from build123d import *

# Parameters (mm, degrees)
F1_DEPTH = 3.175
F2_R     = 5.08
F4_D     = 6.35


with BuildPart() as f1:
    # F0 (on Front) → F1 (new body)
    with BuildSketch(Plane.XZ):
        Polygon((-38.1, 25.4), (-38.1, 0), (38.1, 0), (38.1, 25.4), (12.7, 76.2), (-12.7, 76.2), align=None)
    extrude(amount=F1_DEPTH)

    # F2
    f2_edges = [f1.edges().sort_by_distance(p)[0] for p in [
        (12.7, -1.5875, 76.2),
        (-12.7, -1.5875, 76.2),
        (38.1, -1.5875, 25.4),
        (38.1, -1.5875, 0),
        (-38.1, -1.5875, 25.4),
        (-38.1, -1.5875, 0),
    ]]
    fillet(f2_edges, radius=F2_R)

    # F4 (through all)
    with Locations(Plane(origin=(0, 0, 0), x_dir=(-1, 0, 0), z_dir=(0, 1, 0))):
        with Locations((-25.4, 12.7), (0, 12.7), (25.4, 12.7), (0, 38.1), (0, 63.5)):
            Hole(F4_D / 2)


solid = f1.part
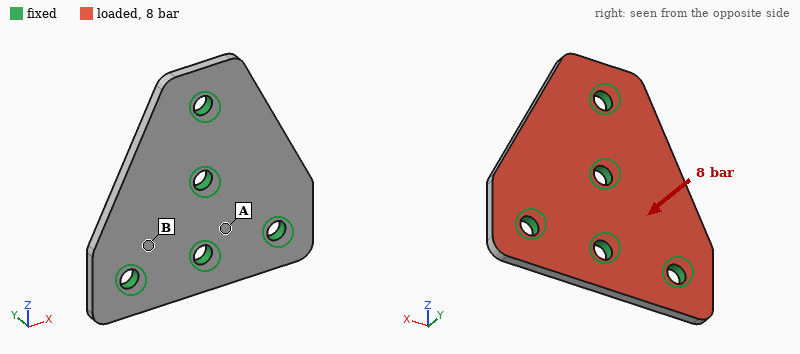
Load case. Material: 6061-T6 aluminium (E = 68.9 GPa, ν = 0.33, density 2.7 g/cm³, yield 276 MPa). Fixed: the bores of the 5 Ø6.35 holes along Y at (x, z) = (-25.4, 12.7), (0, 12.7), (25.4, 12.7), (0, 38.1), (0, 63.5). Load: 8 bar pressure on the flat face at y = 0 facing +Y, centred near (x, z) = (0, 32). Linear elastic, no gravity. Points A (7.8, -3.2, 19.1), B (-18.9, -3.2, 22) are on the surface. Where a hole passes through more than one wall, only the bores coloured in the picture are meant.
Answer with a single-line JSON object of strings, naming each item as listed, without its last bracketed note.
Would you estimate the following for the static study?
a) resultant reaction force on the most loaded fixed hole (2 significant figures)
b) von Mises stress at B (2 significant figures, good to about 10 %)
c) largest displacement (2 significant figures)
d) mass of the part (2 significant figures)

{"resultant reaction force on the most loaded fixed hole": "870 N", "von Mises stress at B": "35 MPa", "largest displacement": "0.12 mm", "mass of the part": "37 g"}
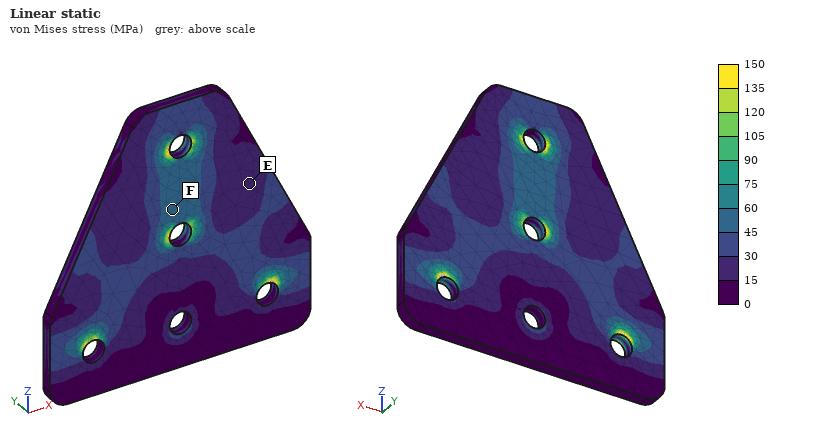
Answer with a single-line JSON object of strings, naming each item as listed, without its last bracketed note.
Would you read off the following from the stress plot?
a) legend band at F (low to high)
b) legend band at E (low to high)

{"legend band at F": "45 to 60 MPa", "legend band at E": "15 to 30 MPa"}
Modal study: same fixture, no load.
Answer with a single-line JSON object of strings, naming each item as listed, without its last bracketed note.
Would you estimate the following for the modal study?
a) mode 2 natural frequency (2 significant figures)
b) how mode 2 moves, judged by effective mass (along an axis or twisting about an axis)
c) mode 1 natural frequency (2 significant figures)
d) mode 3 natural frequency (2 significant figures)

{"mode 2 natural frequency": "6100 Hz", "how mode 2 moves, judged by effective mass": "along Y", "mode 1 natural frequency": "5900 Hz", "mode 3 natural frequency": "11 kHz"}
